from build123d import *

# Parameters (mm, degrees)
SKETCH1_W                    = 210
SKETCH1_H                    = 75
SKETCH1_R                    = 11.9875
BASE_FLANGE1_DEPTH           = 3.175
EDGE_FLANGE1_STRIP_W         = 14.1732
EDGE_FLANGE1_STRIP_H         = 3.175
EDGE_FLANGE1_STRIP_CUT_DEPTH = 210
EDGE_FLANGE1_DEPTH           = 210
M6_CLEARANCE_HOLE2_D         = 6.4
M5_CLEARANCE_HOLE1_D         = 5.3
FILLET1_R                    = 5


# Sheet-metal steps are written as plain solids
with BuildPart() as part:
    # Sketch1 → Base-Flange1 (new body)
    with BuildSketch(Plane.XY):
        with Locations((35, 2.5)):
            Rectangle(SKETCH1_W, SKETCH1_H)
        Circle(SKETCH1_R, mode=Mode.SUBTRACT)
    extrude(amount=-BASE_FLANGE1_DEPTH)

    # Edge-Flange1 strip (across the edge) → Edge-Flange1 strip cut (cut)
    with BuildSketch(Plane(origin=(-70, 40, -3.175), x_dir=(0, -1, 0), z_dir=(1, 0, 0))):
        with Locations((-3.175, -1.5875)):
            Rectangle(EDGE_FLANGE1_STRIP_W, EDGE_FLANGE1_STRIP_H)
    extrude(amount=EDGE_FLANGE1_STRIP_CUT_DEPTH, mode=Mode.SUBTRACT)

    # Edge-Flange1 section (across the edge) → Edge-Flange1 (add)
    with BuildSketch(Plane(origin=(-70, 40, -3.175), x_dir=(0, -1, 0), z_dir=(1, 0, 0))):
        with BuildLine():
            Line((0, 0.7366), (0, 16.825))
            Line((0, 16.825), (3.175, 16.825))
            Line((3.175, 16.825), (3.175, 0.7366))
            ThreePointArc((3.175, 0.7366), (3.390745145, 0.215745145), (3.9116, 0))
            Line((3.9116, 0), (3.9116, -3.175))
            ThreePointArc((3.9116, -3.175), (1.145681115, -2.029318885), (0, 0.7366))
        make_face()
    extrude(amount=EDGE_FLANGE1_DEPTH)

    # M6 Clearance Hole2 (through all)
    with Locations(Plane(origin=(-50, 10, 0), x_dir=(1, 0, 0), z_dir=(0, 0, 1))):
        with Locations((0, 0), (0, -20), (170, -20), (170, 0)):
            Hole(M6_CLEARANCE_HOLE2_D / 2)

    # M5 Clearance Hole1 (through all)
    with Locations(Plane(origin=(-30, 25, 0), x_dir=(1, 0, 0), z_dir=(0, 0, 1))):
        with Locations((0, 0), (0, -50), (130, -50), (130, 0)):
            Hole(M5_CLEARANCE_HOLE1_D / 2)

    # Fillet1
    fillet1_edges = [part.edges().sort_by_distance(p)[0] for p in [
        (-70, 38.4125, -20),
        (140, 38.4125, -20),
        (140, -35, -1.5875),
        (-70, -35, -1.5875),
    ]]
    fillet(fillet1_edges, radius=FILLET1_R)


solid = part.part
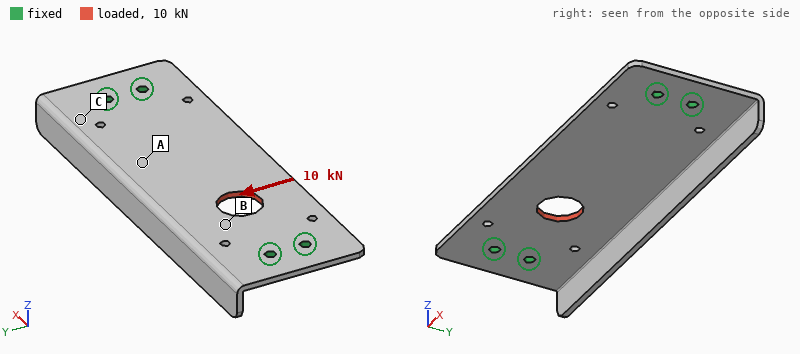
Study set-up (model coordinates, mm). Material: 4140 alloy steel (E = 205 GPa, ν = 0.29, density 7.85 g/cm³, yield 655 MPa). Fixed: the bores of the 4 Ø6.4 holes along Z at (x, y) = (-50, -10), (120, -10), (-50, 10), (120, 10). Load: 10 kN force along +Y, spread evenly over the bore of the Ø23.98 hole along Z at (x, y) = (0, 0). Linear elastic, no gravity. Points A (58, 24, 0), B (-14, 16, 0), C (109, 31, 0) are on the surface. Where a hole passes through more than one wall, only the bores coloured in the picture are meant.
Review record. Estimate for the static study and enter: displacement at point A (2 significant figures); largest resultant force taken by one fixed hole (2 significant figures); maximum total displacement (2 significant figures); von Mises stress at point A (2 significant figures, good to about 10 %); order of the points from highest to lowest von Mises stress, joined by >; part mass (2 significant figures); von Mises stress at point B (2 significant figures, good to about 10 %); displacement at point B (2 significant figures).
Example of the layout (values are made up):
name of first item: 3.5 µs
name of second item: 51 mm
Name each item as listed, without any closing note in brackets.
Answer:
displacement at point A: 44 µm
largest resultant force taken by one fixed hole: 5.2 kN
maximum total displacement: 78 µm
von Mises stress at point A: 28 MPa
order of the points from highest to lowest von Mises stress, joined by >: B > A > C
part mass: 460 g
von Mises stress at point B: 56 MPa
displacement at point B: 36 µm
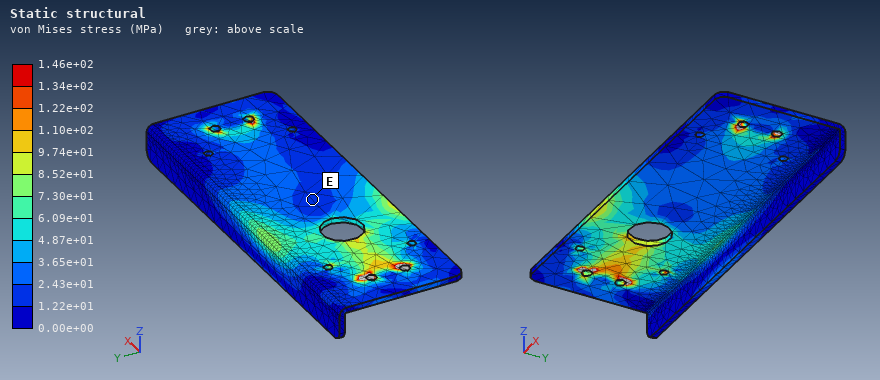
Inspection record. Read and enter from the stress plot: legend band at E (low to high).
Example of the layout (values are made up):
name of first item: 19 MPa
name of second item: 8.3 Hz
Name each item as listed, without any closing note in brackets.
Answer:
legend band at E: 1.22e+01 to 2.43e+01 MPa
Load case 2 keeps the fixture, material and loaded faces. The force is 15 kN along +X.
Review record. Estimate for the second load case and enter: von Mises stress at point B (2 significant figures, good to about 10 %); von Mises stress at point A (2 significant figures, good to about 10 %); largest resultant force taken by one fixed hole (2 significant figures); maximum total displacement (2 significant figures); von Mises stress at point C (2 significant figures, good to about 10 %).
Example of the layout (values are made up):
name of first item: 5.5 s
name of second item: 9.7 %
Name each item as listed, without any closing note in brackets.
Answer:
von Mises stress at point B: 59 MPa
von Mises stress at point A: 21 MPa
largest resultant force taken by one fixed hole: 4.9 kN
maximum total displacement: 18 µm
von Mises stress at point C: 11 MPa
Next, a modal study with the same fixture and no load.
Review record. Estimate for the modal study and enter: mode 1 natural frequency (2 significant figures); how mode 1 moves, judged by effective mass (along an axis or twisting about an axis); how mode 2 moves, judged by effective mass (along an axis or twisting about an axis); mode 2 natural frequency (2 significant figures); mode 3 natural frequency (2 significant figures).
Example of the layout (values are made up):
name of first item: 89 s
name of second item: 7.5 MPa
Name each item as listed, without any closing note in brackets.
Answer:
mode 1 natural frequency: 720 Hz
how mode 1 moves, judged by effective mass: along Z
how mode 2 moves, judged by effective mass: along Z
mode 2 natural frequency: 980 Hz
mode 3 natural frequency: 1600 Hz
